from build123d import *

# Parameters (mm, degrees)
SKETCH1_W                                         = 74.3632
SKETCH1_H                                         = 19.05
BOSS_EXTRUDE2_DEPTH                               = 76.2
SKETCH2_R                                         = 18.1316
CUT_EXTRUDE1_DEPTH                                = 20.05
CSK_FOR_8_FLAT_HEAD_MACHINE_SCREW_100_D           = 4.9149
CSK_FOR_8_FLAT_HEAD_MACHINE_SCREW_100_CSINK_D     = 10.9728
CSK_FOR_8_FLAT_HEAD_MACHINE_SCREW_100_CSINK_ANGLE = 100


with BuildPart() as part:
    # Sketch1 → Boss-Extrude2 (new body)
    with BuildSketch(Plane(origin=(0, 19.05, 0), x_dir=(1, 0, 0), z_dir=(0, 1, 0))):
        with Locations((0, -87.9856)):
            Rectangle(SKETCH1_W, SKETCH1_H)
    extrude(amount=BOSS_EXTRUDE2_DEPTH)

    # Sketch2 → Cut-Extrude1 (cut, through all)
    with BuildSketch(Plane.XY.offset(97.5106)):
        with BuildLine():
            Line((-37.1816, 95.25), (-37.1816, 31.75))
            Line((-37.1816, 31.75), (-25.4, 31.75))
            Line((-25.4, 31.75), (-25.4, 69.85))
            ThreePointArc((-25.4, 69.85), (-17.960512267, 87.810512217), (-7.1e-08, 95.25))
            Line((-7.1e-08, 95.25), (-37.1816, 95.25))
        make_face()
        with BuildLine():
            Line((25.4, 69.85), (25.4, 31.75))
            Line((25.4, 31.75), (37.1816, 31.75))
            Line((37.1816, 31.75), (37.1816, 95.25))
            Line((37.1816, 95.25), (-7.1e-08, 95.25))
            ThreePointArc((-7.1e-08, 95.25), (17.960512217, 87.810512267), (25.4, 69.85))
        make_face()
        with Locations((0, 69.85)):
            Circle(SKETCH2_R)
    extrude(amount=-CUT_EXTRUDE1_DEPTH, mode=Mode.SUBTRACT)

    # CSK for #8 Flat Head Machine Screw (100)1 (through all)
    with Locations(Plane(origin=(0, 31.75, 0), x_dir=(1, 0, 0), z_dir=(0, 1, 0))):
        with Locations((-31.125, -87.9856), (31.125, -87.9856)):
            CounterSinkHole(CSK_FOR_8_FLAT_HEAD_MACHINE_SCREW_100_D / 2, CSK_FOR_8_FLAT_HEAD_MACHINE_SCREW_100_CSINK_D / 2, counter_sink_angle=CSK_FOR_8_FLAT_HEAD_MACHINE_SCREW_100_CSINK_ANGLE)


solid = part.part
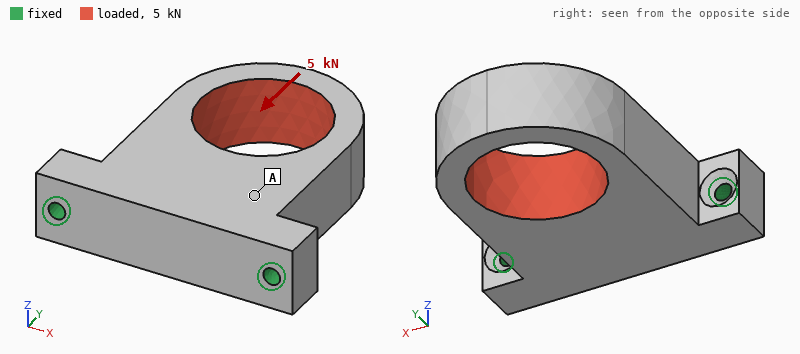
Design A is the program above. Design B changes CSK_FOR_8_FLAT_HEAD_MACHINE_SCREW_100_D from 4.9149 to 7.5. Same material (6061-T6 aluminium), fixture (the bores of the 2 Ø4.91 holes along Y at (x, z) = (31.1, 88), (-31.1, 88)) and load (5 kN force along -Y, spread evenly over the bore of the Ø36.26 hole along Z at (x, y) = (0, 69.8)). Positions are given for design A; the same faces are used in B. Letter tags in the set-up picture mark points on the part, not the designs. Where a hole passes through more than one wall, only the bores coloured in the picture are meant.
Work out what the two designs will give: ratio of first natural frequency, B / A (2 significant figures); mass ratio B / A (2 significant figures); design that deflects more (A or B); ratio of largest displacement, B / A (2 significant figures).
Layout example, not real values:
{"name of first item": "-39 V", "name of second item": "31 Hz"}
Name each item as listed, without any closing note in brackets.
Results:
{"ratio of first natural frequency, B / A": "1.2", "mass ratio B / A": "0.99", "design that deflects more": "A", "ratio of largest displacement, B / A": "0.92"}
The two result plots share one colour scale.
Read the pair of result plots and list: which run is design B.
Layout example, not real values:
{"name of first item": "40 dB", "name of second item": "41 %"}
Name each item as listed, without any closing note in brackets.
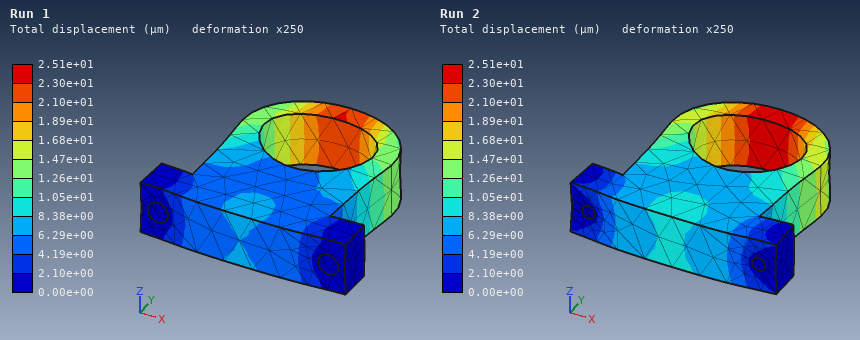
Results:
{"which run is design B": "Run 1"}
